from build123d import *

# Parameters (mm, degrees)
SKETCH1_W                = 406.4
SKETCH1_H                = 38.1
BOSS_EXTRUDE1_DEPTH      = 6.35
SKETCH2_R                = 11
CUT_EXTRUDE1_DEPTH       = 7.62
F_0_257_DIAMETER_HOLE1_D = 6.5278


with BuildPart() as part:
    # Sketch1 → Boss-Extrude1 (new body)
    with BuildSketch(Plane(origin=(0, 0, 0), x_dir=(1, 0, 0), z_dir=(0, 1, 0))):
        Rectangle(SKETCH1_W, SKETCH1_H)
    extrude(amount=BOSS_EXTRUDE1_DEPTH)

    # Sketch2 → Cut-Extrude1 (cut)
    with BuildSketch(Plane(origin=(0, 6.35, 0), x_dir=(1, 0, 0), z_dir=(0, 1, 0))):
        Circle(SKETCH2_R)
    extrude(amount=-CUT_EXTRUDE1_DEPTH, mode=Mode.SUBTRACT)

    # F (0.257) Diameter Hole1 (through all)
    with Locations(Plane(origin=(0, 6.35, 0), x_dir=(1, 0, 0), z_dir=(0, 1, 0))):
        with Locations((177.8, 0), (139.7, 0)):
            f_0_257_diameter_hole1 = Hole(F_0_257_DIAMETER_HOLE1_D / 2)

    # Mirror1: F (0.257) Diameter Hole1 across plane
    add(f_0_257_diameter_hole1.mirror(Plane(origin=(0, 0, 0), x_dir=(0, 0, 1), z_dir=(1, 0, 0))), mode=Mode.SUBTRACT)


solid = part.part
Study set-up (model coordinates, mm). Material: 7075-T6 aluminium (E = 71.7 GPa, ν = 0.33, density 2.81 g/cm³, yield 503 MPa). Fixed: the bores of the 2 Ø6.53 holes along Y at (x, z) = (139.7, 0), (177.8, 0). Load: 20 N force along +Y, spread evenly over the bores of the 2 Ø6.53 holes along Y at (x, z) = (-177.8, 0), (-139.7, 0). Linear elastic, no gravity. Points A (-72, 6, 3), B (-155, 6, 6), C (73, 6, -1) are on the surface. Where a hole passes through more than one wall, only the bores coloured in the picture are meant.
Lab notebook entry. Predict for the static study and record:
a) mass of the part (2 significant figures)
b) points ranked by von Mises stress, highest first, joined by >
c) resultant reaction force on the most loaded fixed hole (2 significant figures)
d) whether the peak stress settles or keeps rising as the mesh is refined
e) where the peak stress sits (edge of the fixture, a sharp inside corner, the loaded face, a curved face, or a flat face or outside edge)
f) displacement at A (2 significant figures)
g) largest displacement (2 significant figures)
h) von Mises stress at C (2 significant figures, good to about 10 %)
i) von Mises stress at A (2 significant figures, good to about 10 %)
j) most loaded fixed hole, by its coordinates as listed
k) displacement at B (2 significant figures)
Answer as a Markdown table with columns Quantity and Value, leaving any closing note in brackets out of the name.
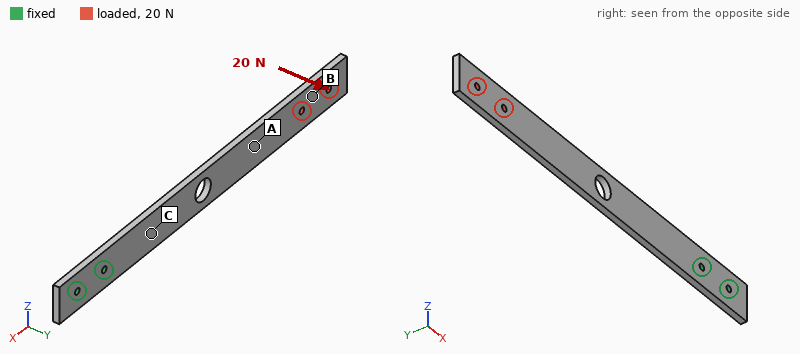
| Quantity | Value |
|---|---|
| mass of the part | 270 g |
| points ranked by von Mises stress, highest first, joined by > | C > A > B |
| resultant reaction force on the most loaded fixed hole | 60 N |
| whether the peak stress settles or keeps rising as the mesh is refined | keeps rising |
| where the peak stress sits | edge of the fixture |
| displacement at A | 1.9 mm |
| largest displacement | 4.0 mm |
| von Mises stress at C | 18 MPa |
| von Mises stress at A | 6.8 MPa |
| most loaded fixed hole, by its coordinates as listed | (139.7, 0) |
| displacement at B | 3.2 mm |
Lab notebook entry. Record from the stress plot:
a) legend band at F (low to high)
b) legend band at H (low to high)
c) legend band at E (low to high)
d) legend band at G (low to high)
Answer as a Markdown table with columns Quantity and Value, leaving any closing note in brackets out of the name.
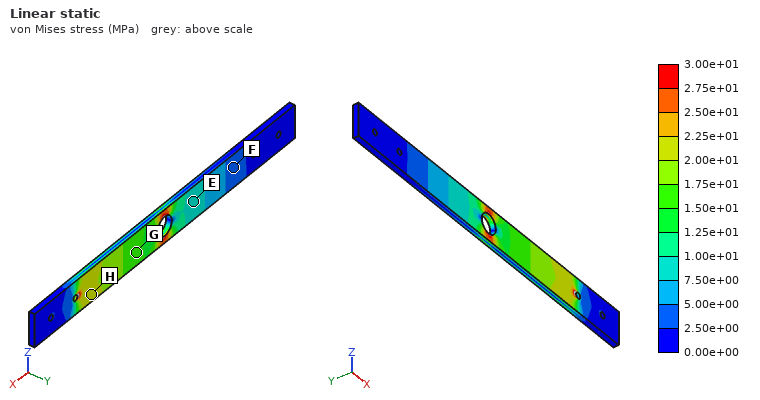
| Quantity | Value |
|---|---|
| legend band at F | 2.50e+00 to 5.00e+00 MPa |
| legend band at H | 2.00e+01 to 2.25e+01 MPa |
| legend band at E | 7.50e+00 to 1.00e+01 MPa |
| legend band at G | 1.50e+01 to 1.75e+01 MPa |
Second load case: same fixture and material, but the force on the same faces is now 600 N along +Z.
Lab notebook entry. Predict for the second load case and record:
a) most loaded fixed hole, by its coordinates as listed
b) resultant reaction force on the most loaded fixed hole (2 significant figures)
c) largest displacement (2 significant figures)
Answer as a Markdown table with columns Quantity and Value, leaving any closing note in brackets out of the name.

| Quantity | Value |
|---|---|
| most loaded fixed hole, by its coordinates as listed | (139.7, 0) |
| resultant reaction force on the most loaded fixed hole | 4.3 kN |
| largest displacement | 3.8 mm |
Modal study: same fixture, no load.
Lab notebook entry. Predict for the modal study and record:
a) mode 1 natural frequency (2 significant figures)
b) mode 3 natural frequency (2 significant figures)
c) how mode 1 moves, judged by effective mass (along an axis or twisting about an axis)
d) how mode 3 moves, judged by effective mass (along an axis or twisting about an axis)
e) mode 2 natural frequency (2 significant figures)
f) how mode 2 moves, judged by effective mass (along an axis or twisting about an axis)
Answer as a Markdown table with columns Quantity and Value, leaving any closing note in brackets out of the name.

| Quantity | Value |
|---|---|
| mode 1 natural frequency | 43 Hz |
| mode 3 natural frequency | 270 Hz |
| how mode 1 moves, judged by effective mass | along Y |
| how mode 3 moves, judged by effective mass | along Y |
| mode 2 natural frequency | 240 Hz |
| how mode 2 moves, judged by effective mass | along Z |
